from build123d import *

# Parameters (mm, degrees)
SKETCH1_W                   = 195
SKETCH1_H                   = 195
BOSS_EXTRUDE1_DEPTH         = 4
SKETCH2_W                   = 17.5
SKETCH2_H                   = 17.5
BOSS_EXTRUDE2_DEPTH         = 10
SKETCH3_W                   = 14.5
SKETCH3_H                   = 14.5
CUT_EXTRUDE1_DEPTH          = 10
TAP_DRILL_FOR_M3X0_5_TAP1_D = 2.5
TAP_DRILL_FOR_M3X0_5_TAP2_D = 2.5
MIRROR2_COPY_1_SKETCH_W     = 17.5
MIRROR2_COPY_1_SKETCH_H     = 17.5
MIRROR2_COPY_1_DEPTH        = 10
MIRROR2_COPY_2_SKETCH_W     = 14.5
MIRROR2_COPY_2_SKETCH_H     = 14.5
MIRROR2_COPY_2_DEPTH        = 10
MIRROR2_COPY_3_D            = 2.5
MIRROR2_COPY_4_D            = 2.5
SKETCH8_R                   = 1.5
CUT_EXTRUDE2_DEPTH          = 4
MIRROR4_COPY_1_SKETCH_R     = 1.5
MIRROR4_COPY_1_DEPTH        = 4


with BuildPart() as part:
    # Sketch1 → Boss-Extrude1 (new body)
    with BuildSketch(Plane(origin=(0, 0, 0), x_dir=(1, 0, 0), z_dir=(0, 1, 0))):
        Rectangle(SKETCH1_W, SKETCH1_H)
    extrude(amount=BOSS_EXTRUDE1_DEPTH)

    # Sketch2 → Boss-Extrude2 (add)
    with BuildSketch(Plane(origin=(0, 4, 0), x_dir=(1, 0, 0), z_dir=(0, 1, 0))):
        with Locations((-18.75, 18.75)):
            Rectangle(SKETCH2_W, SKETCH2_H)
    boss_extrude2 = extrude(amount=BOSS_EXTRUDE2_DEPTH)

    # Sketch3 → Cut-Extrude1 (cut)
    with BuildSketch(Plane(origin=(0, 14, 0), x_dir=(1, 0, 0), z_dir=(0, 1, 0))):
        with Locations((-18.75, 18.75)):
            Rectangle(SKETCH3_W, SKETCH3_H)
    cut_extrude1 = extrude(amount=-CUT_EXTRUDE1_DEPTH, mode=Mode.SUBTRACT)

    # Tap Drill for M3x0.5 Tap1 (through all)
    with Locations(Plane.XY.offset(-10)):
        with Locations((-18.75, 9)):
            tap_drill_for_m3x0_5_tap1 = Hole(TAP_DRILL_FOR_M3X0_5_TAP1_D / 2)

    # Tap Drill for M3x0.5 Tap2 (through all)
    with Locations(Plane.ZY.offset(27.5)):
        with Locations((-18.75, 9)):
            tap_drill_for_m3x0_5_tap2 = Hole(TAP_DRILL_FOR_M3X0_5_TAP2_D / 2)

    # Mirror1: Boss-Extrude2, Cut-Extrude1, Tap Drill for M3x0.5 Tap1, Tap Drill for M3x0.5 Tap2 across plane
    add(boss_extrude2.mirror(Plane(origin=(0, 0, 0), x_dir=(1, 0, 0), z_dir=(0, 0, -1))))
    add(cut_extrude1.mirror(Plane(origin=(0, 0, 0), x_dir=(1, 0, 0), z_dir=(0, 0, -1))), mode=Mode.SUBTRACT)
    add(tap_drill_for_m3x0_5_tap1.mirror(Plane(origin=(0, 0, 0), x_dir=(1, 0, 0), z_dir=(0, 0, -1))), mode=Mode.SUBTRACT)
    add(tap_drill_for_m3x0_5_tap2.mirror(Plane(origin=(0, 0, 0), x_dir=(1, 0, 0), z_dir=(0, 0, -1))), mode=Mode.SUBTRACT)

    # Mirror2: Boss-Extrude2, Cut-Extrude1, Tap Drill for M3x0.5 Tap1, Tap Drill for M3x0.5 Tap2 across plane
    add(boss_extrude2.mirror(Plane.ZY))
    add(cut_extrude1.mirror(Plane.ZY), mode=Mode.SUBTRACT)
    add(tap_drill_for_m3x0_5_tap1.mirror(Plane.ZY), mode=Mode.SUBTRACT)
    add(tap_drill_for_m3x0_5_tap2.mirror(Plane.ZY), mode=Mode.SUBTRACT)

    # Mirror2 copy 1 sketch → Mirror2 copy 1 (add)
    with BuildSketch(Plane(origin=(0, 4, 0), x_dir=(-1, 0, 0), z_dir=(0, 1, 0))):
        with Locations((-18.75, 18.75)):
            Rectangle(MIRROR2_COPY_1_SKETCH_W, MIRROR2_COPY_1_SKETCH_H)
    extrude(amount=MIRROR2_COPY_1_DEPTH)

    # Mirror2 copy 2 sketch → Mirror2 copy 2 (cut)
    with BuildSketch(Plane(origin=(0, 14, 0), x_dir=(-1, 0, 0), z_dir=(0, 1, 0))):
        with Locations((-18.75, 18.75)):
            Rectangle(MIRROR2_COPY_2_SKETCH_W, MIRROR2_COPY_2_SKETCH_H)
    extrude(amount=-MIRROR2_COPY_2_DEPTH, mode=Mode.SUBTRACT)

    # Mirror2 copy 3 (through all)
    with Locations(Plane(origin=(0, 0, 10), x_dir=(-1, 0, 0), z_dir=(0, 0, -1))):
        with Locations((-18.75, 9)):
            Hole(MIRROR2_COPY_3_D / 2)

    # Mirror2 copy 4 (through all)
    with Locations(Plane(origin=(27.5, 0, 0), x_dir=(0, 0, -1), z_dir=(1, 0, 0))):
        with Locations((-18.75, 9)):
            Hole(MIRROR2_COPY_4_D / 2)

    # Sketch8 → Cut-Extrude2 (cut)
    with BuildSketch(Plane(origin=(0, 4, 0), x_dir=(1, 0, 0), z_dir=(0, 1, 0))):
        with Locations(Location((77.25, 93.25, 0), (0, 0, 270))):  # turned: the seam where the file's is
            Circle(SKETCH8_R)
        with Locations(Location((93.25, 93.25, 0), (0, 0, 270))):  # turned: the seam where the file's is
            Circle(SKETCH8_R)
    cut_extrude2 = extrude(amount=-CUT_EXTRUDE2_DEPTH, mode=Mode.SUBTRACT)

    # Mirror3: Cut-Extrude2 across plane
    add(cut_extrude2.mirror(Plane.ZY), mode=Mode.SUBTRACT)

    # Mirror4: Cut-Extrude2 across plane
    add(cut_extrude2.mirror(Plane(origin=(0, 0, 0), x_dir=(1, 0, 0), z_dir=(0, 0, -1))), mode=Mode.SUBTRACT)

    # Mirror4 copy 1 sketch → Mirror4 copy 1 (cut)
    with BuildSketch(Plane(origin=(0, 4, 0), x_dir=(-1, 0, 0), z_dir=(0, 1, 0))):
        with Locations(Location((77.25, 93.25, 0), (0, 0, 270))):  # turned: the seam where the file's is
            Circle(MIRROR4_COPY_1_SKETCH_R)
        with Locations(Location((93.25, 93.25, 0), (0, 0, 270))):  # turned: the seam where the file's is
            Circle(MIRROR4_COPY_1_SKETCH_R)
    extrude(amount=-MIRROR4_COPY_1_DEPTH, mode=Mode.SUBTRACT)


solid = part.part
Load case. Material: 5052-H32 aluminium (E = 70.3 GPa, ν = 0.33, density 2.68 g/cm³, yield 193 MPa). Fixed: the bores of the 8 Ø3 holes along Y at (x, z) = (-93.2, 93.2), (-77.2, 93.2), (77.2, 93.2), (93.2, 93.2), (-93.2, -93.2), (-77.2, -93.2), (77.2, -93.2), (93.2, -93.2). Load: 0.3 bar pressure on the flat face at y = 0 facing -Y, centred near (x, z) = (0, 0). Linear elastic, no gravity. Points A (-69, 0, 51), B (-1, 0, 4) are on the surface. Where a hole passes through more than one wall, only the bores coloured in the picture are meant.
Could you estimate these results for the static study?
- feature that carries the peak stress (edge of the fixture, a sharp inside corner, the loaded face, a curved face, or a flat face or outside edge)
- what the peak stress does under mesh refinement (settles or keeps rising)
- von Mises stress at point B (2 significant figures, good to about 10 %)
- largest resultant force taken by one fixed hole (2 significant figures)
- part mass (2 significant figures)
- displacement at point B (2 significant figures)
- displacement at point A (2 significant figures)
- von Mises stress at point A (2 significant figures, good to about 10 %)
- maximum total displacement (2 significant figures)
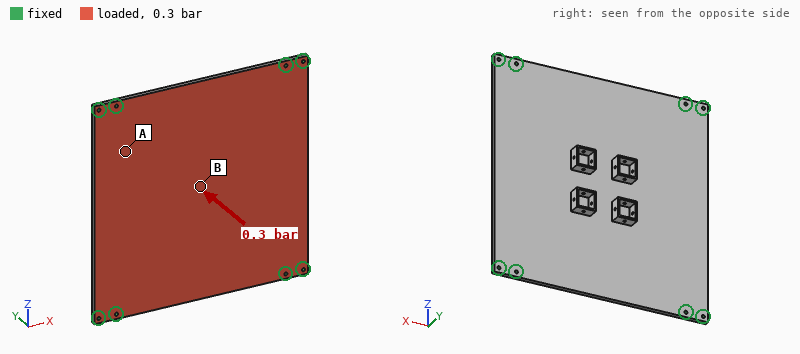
edge of the fixture
keeps rising
22 MPa
370 N
420 g
0.57 mm
0.26 mm
9.4 MPa
0.57 mm
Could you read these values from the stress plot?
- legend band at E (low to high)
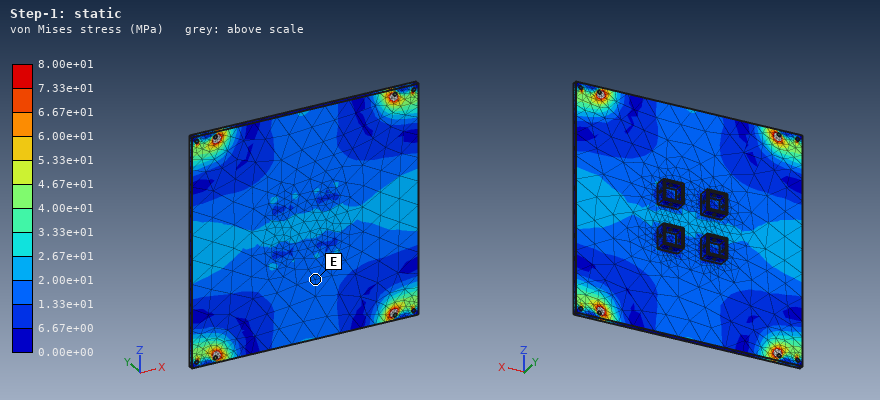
1.33e+01 to 2.00e+01 MPa
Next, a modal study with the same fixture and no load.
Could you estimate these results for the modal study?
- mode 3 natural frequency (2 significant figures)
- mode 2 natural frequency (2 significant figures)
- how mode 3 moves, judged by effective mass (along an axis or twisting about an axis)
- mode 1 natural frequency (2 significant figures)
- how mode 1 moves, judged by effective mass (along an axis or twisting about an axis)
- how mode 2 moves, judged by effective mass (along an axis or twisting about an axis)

840 Hz
670 Hz
twisting about X
410 Hz
along Y
twisting about Z
